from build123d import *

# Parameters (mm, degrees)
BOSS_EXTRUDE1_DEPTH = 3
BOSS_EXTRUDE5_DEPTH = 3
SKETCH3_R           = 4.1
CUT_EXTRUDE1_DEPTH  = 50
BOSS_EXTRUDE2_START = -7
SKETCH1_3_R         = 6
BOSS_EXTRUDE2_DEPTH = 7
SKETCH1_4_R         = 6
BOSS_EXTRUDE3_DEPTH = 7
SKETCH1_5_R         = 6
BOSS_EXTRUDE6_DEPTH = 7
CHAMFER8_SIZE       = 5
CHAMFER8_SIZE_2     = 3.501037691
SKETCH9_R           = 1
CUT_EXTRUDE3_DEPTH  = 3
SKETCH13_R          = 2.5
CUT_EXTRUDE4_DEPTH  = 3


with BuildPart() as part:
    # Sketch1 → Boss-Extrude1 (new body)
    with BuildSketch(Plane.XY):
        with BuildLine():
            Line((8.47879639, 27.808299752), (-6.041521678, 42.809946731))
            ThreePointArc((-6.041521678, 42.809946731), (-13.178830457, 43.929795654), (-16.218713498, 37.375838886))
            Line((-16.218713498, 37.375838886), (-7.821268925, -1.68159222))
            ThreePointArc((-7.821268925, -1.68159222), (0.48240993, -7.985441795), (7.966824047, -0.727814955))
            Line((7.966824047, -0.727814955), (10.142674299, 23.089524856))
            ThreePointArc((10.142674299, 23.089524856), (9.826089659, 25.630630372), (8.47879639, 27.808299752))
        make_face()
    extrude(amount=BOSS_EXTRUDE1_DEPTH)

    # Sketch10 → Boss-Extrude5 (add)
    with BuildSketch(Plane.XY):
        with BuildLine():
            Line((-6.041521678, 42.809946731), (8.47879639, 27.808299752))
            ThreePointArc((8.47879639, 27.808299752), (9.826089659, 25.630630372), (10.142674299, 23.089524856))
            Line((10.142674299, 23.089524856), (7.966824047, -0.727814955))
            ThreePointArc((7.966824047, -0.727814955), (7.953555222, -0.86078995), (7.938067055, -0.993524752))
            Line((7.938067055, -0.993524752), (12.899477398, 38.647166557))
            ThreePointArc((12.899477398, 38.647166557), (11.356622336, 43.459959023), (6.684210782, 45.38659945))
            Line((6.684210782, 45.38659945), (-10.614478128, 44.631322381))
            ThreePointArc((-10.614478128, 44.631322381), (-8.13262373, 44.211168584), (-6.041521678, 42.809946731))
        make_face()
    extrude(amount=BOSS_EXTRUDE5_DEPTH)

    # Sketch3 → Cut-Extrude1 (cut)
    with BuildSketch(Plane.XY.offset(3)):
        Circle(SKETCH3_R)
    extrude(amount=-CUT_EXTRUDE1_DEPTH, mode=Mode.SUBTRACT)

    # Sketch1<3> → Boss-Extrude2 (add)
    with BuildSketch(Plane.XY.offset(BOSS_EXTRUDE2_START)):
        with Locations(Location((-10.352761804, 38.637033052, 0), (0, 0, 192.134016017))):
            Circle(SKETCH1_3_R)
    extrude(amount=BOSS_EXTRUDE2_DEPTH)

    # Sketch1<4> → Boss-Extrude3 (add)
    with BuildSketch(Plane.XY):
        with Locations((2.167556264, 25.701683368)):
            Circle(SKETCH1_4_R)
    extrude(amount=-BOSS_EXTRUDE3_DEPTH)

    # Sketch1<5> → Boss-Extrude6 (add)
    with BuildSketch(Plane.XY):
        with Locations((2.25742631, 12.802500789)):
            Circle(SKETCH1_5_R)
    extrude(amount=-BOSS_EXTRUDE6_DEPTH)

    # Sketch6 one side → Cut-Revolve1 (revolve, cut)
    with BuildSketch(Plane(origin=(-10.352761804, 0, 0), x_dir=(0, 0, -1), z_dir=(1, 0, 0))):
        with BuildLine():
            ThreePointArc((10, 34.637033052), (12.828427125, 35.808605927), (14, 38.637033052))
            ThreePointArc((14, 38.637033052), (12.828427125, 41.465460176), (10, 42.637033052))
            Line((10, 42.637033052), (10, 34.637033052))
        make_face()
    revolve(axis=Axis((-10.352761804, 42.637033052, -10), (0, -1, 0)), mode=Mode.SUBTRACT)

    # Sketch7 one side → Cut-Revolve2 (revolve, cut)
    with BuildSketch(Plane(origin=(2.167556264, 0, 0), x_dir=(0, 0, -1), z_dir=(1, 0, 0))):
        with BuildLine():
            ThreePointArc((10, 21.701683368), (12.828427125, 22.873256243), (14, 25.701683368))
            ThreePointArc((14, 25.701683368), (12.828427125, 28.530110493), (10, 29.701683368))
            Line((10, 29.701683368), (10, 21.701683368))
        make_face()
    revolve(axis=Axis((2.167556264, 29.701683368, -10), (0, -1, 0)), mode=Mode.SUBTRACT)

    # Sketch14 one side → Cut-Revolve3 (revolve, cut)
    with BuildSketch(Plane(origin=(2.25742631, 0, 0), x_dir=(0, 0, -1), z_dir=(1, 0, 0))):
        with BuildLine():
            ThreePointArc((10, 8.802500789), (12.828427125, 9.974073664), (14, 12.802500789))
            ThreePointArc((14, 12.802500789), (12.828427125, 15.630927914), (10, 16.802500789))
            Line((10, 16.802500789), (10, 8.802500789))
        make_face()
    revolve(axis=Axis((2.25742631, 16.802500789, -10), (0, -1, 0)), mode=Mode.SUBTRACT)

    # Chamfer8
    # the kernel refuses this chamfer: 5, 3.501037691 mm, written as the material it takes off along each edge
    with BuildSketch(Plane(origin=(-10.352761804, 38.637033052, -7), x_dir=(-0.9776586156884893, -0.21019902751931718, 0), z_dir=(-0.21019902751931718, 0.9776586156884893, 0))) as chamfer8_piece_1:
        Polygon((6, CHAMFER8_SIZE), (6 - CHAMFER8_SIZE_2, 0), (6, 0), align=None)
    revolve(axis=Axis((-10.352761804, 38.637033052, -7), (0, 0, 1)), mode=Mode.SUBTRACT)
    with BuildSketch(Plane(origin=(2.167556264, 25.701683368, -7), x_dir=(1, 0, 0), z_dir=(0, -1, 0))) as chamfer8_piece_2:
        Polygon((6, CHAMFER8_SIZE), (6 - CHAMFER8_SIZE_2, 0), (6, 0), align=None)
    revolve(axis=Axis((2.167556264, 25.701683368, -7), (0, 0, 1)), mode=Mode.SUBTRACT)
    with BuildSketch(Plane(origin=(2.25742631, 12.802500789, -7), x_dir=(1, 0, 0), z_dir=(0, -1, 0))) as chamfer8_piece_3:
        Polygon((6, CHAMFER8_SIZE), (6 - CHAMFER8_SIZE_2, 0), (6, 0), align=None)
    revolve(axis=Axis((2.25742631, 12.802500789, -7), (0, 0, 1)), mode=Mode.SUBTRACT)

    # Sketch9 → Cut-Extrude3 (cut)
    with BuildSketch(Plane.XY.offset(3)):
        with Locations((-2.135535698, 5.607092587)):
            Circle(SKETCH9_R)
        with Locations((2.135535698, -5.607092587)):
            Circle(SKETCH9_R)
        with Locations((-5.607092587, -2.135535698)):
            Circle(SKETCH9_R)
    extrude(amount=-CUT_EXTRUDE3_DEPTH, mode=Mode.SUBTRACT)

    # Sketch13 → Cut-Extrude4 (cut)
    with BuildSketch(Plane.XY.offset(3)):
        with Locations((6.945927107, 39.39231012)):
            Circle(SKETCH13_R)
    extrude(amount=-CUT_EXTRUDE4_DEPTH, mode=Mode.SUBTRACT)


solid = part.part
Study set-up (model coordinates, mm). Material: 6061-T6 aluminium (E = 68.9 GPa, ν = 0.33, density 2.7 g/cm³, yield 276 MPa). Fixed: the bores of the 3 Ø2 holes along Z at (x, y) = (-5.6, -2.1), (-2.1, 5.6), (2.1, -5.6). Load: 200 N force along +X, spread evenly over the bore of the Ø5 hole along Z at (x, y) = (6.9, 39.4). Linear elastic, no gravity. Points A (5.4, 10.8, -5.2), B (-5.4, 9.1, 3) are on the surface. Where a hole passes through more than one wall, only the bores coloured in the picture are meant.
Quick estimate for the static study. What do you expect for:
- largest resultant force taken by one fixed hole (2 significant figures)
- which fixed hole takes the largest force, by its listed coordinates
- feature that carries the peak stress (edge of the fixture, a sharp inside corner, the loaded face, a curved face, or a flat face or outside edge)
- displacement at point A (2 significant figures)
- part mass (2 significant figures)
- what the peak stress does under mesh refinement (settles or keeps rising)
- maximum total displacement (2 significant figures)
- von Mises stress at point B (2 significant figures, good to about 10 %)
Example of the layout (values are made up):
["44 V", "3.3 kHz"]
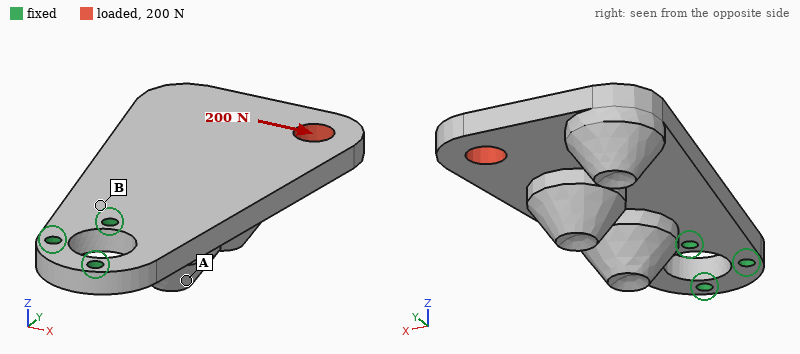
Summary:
["480 N", "(-2.1, 5.6)", "edge of the fixture", "11 µm", "13 g", "keeps rising", "64 µm", "19 MPa"]
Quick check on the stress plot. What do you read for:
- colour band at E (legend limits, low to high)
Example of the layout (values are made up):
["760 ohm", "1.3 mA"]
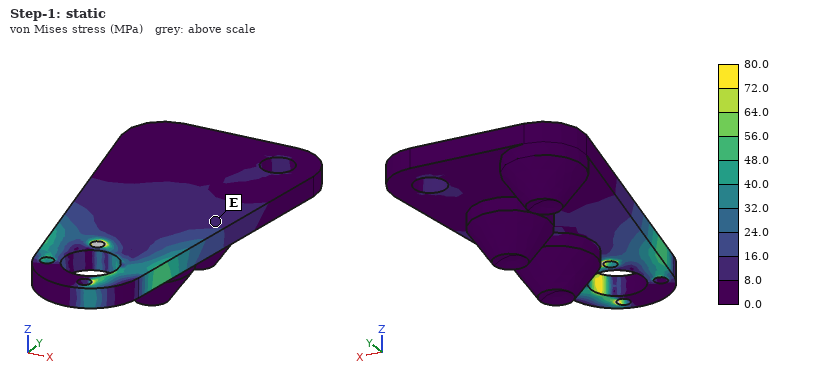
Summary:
["8.0 to 16.0 MPa"]
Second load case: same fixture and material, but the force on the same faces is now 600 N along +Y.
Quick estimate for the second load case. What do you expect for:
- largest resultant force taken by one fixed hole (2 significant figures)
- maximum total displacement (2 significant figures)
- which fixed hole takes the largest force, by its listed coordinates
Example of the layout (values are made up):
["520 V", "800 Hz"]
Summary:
["480 N", "56 µm", "(-2.1, 5.6)"]
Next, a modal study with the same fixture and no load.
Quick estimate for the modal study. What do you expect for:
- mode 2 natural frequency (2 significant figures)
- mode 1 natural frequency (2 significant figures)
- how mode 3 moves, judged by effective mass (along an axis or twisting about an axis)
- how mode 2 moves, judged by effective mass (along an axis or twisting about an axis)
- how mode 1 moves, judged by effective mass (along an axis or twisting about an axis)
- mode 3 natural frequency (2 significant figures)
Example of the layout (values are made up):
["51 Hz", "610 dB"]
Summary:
["3700 Hz", "1300 Hz", "along X", "along X", "along Z", "4200 Hz"]
